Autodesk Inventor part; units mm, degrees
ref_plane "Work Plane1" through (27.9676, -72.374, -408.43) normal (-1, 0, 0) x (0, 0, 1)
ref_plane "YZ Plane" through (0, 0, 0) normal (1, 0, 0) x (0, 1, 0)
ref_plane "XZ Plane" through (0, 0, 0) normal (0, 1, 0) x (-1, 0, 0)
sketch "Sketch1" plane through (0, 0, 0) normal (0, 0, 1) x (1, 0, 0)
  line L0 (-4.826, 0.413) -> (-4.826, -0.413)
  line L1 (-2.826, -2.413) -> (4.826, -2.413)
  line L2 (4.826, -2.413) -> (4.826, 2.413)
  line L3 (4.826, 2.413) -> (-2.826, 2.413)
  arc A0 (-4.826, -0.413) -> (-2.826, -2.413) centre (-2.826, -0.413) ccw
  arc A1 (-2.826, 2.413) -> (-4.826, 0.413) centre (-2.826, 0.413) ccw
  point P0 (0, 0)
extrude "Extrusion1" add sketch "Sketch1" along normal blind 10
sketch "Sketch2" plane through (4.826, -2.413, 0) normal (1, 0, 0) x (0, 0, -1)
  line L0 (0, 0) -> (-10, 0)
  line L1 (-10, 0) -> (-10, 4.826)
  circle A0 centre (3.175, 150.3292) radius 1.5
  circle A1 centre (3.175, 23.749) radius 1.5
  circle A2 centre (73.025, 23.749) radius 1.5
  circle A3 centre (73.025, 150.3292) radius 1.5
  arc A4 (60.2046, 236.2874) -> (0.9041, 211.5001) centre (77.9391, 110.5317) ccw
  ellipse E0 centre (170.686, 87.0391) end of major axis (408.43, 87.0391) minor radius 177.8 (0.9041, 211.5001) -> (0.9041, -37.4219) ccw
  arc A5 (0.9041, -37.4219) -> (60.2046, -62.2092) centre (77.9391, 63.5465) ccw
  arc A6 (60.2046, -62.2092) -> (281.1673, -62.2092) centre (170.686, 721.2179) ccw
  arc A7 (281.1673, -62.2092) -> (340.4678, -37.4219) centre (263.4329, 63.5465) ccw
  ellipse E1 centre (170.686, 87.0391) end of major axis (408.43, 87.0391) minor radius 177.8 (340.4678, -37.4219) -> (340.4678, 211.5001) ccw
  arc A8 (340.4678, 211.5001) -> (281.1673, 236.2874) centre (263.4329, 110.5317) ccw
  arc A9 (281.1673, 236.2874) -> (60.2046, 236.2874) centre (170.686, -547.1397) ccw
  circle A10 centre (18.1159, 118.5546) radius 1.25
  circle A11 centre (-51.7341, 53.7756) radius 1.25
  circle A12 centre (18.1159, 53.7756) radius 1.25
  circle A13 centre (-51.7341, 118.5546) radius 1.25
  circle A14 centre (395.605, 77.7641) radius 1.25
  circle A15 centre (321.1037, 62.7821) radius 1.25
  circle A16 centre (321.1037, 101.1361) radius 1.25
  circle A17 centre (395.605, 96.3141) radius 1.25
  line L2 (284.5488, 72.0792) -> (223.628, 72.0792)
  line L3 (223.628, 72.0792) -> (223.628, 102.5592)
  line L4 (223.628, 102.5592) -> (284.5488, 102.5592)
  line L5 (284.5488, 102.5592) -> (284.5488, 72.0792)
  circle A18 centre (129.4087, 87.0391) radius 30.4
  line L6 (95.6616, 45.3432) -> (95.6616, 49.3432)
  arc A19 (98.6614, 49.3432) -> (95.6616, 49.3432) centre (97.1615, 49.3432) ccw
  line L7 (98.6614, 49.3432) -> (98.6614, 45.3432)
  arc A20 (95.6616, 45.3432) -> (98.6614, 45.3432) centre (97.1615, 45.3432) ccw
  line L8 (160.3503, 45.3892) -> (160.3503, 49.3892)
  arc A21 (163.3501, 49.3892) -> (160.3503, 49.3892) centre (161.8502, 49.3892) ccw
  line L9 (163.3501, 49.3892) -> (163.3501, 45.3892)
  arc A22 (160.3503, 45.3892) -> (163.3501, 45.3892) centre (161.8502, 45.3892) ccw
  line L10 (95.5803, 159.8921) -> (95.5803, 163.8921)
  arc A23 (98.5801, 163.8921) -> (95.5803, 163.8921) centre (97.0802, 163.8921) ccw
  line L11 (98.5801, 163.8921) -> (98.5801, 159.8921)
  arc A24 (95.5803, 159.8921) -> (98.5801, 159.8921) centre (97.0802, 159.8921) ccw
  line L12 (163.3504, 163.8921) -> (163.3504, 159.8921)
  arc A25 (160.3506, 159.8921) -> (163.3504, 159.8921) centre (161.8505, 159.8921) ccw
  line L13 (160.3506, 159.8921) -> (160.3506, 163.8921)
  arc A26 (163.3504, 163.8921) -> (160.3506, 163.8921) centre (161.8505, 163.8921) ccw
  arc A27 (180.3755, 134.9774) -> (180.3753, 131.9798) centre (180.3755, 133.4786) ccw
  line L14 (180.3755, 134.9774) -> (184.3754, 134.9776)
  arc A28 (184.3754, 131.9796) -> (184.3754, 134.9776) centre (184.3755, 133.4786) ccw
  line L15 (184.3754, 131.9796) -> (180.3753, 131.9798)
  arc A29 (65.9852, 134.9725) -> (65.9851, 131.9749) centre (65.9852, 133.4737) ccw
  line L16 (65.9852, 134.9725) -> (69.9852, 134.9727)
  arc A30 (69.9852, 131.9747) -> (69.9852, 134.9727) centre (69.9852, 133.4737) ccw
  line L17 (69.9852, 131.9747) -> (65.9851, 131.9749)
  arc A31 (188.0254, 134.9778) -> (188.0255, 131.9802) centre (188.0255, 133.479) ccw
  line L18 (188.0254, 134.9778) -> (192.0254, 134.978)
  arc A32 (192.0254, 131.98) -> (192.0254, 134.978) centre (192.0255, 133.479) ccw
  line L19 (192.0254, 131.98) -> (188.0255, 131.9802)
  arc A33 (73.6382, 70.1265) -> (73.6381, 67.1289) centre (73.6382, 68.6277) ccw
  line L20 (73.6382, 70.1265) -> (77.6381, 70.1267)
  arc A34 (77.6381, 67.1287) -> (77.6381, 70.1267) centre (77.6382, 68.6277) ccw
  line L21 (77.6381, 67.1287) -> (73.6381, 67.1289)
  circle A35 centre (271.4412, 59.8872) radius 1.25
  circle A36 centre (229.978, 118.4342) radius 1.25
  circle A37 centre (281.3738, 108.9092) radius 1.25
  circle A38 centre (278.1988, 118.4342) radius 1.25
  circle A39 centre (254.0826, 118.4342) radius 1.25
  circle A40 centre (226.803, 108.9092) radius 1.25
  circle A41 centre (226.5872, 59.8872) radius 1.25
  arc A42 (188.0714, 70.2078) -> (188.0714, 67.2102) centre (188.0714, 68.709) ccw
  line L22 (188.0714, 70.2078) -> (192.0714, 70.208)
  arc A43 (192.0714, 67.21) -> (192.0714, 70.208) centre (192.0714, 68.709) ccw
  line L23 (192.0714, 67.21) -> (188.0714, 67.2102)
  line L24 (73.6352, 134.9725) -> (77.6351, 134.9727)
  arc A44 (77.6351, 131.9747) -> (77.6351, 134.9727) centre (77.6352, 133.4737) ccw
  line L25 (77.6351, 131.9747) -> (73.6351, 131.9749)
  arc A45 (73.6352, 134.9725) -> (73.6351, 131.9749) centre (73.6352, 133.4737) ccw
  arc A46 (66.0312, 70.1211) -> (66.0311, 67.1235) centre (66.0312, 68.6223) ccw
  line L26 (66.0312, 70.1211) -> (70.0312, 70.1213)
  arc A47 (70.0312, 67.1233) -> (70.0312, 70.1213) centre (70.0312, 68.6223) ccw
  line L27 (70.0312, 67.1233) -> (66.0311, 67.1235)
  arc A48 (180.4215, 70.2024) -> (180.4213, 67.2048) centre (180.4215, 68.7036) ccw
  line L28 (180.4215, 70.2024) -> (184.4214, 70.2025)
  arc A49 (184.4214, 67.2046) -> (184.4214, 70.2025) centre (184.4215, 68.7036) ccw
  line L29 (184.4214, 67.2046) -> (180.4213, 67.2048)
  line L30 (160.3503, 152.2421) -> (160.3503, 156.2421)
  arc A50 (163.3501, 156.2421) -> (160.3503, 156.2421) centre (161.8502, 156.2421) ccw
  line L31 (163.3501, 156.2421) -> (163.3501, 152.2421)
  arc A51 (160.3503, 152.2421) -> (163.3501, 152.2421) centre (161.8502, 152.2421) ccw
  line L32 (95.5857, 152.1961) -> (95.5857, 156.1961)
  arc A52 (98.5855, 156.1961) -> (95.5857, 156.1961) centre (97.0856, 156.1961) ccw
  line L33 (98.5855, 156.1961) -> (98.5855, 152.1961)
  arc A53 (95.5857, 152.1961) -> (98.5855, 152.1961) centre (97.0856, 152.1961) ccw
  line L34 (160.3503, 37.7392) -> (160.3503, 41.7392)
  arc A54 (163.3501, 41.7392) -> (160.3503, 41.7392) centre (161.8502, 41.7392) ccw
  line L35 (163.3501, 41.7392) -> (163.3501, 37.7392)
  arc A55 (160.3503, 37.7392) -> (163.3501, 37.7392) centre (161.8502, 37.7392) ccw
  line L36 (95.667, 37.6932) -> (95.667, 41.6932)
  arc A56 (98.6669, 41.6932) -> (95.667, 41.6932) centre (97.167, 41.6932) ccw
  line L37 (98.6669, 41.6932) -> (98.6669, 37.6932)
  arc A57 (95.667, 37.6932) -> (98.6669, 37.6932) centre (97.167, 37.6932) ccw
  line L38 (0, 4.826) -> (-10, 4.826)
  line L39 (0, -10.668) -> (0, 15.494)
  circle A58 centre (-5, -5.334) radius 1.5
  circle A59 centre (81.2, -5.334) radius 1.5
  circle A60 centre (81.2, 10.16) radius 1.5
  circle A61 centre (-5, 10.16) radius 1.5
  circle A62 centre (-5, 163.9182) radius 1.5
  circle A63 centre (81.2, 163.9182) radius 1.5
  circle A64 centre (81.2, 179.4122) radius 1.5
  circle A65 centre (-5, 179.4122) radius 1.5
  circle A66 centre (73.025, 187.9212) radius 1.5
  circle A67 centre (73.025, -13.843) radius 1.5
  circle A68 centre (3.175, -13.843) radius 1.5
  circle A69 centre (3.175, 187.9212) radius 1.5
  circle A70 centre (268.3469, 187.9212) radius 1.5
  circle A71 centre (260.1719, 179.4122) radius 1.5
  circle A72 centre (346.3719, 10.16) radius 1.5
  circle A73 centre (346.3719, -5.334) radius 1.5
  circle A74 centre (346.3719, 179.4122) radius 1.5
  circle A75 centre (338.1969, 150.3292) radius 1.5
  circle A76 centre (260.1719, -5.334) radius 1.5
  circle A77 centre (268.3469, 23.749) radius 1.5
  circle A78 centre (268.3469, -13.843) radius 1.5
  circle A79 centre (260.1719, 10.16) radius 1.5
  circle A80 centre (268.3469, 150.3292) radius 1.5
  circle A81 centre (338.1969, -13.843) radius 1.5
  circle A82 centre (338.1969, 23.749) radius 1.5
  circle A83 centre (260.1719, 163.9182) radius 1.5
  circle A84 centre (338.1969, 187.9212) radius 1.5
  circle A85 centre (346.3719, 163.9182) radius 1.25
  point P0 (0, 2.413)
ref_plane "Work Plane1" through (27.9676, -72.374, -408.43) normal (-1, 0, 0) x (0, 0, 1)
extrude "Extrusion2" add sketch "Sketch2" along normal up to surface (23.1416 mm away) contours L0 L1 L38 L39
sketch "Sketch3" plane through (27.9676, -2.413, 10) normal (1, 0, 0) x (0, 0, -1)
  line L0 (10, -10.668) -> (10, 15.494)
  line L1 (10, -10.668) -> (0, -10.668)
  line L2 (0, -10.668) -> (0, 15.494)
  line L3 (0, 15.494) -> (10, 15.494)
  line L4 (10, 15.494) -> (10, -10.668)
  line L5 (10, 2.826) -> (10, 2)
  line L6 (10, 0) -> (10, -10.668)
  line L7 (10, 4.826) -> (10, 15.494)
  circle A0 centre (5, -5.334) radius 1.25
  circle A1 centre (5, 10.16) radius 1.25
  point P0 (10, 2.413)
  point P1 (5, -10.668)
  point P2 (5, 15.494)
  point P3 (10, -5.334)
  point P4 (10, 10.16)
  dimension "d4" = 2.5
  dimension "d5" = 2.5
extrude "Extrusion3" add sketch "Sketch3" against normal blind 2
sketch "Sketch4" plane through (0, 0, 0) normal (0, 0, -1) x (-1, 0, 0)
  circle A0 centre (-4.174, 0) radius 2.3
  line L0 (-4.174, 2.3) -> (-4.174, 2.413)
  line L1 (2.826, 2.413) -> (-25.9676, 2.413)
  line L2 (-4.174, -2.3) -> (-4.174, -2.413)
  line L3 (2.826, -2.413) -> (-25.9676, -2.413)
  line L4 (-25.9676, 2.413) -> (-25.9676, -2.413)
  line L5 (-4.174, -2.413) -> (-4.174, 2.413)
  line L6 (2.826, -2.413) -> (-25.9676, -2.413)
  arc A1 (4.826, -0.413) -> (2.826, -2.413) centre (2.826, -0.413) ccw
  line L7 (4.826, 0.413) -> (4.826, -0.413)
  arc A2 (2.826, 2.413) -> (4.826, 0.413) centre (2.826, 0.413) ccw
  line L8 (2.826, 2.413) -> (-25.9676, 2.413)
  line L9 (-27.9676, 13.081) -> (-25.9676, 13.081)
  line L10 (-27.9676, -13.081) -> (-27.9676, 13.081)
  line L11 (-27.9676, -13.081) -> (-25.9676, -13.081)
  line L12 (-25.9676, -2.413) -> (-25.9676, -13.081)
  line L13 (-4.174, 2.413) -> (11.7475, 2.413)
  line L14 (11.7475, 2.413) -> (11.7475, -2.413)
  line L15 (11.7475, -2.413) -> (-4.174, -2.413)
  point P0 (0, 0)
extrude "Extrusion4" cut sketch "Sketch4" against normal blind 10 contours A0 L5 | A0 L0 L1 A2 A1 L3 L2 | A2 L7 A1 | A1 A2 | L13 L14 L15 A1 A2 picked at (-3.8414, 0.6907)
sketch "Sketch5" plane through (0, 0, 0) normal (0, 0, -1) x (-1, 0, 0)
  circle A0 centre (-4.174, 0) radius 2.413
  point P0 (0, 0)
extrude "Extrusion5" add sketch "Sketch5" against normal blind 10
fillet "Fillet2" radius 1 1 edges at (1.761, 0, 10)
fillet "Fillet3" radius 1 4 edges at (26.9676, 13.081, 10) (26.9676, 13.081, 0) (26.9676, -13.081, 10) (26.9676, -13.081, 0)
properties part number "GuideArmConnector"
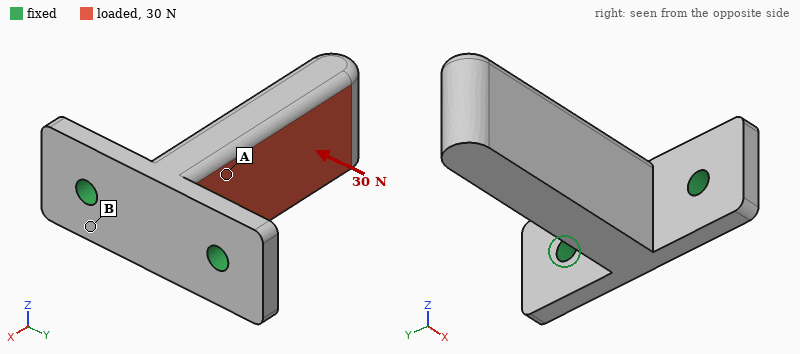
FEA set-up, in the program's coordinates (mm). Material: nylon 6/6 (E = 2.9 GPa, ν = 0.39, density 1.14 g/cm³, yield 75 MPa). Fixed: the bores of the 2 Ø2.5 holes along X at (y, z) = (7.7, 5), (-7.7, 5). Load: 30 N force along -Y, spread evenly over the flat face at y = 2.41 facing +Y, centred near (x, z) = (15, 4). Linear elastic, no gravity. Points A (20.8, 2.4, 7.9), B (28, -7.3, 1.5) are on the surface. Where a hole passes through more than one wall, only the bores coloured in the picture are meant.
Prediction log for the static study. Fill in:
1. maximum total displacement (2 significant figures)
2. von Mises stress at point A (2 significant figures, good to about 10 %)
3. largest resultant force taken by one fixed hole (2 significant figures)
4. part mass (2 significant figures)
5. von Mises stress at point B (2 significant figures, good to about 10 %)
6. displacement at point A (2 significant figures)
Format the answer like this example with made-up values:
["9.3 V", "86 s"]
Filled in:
["0.39 mm", "5.1 MPa", "36 N", "1.9 g", "2.4 MPa", "0.076 mm"]
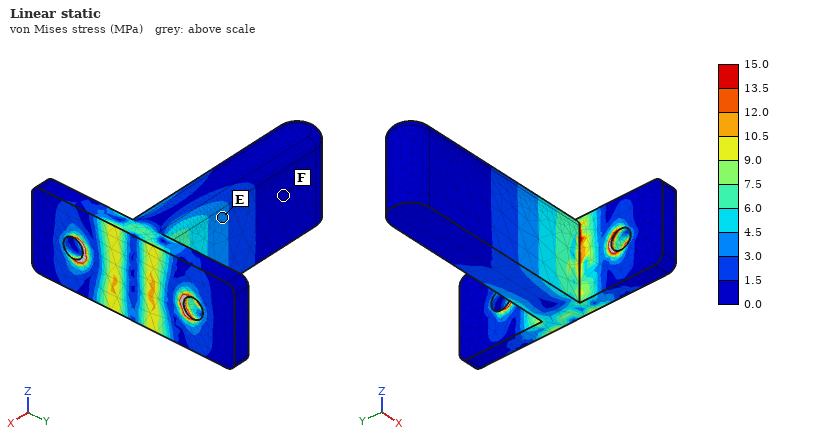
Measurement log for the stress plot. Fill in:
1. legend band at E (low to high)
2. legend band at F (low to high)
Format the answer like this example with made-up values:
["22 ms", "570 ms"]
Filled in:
["3.0 to 4.5 MPa", "0.0 to 1.5 MPa"]
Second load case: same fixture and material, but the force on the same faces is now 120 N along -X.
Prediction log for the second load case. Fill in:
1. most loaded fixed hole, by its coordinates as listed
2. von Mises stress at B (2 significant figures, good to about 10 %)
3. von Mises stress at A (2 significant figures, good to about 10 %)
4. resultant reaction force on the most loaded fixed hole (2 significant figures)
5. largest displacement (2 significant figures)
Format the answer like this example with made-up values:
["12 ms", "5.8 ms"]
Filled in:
["(7.7, 5)", "7.8 MPa", "7.4 MPa", "89 N", "0.41 mm"]
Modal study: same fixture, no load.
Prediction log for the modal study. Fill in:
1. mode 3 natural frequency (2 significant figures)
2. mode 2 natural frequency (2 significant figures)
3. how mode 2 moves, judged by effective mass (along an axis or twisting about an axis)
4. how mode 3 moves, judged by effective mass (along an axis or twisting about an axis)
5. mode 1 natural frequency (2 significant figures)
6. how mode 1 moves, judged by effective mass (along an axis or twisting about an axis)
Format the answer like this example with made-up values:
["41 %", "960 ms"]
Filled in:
["5100 Hz", "1500 Hz", "along Y", "along X", "1100 Hz", "along Z"]
